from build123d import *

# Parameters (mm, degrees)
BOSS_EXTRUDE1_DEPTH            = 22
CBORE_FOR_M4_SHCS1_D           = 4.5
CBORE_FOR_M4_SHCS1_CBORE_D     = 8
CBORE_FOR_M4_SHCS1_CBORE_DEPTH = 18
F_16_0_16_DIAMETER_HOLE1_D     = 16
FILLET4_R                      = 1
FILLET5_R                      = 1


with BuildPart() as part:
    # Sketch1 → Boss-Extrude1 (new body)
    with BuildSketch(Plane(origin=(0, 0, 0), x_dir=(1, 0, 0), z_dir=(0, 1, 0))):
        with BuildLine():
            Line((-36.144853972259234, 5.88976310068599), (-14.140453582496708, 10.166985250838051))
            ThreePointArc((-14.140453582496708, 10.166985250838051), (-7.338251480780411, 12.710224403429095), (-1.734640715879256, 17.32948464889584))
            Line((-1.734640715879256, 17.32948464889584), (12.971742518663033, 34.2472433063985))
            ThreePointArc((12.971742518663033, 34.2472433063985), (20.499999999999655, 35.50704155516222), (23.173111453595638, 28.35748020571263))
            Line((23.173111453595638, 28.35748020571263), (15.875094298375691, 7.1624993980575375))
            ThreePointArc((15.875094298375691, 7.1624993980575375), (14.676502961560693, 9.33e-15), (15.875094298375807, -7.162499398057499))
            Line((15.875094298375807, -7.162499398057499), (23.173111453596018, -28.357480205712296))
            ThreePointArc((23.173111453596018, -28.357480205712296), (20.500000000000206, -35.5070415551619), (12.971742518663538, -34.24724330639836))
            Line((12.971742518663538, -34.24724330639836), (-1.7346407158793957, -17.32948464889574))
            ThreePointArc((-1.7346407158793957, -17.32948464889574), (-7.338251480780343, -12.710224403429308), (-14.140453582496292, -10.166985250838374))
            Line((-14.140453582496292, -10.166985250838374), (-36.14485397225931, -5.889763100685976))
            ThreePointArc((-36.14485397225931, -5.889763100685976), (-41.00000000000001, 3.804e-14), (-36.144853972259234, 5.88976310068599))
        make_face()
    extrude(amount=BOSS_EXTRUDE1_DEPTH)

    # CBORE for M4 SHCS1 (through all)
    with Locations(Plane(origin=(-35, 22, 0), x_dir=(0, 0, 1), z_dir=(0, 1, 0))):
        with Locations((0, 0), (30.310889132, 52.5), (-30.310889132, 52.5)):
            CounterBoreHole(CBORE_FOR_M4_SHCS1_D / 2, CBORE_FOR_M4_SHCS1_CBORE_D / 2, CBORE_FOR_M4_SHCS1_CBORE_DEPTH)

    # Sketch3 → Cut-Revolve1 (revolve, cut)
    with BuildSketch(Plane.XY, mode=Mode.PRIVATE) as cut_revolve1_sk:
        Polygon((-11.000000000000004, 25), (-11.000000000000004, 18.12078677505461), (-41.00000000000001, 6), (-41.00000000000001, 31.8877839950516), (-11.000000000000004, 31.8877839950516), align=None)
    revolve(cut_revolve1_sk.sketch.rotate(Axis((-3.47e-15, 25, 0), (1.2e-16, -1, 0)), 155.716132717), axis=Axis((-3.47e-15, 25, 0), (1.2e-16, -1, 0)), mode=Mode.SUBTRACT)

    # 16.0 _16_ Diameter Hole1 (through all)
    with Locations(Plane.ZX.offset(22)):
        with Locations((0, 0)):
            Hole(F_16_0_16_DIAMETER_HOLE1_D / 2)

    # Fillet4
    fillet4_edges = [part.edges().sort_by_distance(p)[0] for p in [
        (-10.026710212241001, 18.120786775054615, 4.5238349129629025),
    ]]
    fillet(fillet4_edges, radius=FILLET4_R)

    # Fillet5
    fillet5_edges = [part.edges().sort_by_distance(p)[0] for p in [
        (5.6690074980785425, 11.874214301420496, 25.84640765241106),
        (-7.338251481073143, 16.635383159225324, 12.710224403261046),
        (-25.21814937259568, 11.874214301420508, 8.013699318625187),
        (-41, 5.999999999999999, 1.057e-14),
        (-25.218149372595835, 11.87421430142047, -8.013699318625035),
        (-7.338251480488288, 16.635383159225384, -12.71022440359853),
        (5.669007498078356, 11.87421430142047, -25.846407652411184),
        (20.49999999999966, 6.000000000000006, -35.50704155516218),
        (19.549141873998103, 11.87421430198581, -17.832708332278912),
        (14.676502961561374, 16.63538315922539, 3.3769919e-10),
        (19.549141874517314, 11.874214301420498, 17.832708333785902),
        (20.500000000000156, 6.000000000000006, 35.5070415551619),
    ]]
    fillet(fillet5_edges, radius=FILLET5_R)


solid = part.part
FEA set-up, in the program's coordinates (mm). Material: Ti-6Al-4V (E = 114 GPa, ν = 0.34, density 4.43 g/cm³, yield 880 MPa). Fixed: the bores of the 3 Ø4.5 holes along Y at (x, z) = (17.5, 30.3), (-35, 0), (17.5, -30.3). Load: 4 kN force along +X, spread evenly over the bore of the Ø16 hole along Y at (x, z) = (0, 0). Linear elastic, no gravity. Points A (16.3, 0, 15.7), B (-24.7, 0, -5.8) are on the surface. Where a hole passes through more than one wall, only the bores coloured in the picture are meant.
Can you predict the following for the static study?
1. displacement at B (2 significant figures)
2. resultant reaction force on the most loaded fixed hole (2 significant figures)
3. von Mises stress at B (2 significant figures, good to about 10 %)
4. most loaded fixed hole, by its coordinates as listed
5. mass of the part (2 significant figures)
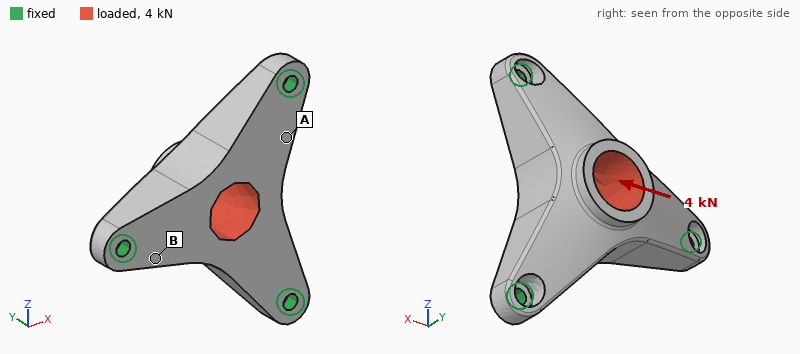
2.9 µm
2.4 kN
18 MPa
(-35, 0)
100 g
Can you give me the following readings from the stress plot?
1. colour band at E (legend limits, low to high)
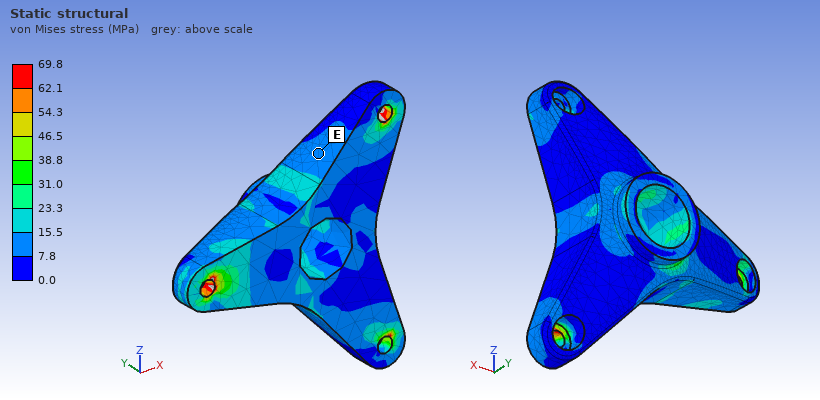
7.8 to 15.5 MPa
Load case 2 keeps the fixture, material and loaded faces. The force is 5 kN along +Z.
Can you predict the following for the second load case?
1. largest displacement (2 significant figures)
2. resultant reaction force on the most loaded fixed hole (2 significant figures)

12 µm
2.7 kN
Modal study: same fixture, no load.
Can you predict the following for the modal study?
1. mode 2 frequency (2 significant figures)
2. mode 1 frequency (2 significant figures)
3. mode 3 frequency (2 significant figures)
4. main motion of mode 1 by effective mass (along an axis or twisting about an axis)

15 kHz
10 kHz
15 kHz
along Y
